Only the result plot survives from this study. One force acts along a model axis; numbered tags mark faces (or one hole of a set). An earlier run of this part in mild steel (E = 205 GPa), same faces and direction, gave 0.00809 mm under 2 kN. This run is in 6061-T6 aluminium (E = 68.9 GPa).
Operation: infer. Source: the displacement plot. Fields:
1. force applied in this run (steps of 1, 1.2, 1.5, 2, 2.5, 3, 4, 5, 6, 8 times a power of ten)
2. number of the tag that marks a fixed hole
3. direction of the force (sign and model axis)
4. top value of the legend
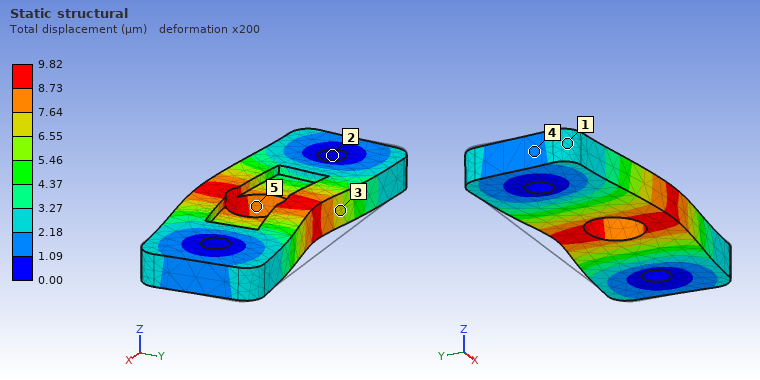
800 N
2
-Y
9.82 µm
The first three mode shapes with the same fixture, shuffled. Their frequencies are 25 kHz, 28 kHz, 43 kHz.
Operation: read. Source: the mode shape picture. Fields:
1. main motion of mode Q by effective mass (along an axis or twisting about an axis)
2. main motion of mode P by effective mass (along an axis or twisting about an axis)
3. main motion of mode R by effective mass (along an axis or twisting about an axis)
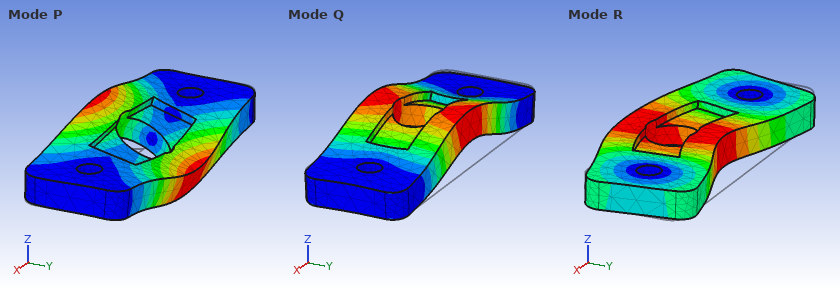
along Z
twisting about X
along Y
